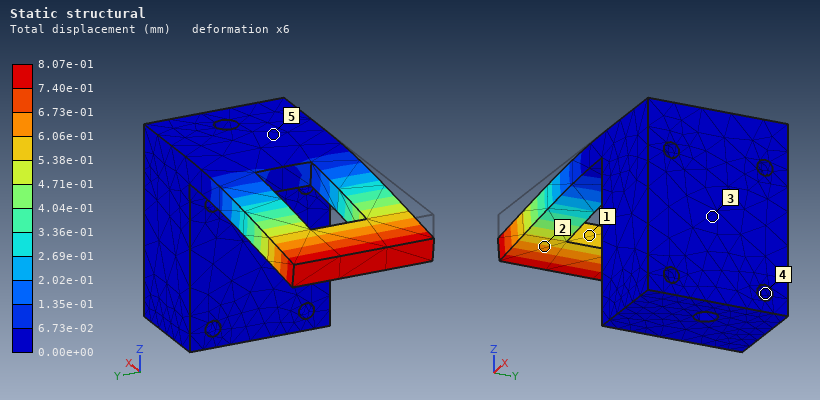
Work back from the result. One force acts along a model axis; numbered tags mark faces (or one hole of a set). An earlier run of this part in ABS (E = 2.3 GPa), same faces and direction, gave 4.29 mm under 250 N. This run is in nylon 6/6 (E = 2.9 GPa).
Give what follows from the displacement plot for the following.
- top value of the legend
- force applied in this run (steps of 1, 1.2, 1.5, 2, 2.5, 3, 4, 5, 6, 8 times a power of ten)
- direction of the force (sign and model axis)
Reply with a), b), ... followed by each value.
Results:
a) 8.07e-01 mm
b) 60 N
c) -Z
